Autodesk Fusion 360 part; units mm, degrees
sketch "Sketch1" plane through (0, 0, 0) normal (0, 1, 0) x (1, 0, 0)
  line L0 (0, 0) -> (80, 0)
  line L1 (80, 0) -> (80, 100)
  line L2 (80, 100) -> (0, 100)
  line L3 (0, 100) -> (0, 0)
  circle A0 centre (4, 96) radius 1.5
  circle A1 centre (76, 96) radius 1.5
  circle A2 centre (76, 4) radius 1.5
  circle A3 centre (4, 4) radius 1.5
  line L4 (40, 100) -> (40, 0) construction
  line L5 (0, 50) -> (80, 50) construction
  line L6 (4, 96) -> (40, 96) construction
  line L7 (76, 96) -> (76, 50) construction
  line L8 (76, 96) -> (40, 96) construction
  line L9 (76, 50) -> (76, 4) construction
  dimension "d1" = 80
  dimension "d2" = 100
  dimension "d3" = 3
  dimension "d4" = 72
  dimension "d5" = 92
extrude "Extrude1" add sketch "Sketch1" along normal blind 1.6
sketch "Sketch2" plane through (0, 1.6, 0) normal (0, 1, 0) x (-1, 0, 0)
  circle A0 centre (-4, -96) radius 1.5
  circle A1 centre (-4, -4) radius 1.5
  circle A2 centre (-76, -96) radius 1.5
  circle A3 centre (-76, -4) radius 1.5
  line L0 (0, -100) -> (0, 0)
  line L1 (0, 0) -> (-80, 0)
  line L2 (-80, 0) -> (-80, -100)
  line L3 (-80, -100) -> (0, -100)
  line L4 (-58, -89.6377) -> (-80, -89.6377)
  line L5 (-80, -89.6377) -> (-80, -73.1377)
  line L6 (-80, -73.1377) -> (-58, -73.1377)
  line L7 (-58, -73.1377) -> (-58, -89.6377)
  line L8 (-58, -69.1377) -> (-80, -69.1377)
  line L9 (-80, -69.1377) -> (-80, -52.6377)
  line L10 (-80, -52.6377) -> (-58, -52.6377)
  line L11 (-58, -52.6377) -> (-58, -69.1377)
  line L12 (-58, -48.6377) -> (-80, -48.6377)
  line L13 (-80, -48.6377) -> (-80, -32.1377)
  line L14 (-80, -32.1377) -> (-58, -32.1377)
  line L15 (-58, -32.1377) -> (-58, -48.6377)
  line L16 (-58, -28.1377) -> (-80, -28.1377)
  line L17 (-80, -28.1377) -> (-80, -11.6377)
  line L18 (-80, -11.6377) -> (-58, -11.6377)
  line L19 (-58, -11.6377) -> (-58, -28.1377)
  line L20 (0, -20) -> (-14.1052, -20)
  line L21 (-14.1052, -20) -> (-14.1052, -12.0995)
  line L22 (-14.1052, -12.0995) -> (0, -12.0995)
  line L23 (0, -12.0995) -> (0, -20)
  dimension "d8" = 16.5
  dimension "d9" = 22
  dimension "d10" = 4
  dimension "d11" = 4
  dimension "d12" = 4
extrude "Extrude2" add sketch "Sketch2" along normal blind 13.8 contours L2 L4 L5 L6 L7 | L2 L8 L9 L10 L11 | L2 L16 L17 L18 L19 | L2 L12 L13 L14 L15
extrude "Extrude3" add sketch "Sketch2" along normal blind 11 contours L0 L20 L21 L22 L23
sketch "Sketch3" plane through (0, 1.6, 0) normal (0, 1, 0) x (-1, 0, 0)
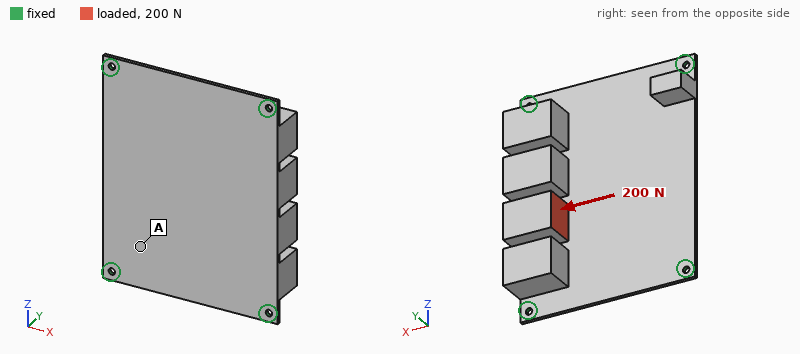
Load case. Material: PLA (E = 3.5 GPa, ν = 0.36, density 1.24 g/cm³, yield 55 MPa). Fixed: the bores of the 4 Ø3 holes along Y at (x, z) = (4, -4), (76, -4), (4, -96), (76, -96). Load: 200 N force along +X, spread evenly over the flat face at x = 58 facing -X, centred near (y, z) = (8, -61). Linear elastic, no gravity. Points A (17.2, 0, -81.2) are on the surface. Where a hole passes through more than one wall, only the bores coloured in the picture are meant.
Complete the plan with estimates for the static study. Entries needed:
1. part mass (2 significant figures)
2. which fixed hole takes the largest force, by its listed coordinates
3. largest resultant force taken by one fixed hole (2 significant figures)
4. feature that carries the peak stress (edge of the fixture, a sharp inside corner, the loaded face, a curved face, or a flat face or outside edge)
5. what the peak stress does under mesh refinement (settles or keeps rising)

42 g
(76, -96)
80 N
edge of the fixture
keeps rising
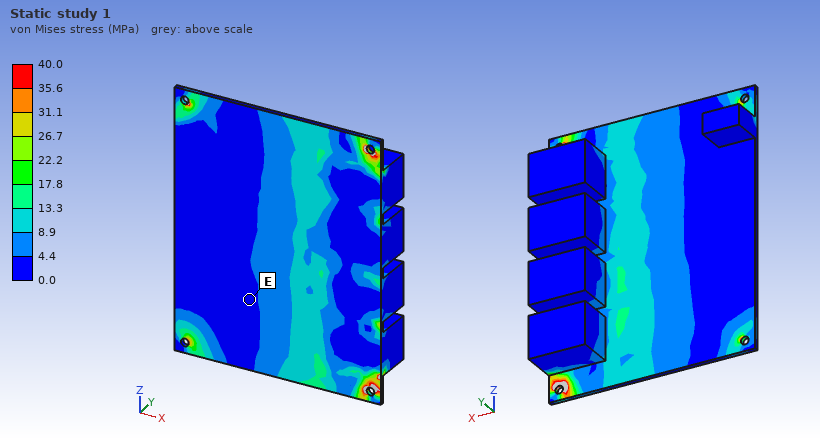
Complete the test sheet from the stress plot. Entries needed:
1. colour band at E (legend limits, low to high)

0.0 to 4.4 MPa
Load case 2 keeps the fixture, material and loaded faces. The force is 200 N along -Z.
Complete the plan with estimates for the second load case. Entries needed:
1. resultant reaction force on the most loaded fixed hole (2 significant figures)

86 N
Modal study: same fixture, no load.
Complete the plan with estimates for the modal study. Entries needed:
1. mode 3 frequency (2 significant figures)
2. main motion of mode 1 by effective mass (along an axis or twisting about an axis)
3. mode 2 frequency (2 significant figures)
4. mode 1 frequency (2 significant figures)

450 Hz
along Y
330 Hz
180 Hz
